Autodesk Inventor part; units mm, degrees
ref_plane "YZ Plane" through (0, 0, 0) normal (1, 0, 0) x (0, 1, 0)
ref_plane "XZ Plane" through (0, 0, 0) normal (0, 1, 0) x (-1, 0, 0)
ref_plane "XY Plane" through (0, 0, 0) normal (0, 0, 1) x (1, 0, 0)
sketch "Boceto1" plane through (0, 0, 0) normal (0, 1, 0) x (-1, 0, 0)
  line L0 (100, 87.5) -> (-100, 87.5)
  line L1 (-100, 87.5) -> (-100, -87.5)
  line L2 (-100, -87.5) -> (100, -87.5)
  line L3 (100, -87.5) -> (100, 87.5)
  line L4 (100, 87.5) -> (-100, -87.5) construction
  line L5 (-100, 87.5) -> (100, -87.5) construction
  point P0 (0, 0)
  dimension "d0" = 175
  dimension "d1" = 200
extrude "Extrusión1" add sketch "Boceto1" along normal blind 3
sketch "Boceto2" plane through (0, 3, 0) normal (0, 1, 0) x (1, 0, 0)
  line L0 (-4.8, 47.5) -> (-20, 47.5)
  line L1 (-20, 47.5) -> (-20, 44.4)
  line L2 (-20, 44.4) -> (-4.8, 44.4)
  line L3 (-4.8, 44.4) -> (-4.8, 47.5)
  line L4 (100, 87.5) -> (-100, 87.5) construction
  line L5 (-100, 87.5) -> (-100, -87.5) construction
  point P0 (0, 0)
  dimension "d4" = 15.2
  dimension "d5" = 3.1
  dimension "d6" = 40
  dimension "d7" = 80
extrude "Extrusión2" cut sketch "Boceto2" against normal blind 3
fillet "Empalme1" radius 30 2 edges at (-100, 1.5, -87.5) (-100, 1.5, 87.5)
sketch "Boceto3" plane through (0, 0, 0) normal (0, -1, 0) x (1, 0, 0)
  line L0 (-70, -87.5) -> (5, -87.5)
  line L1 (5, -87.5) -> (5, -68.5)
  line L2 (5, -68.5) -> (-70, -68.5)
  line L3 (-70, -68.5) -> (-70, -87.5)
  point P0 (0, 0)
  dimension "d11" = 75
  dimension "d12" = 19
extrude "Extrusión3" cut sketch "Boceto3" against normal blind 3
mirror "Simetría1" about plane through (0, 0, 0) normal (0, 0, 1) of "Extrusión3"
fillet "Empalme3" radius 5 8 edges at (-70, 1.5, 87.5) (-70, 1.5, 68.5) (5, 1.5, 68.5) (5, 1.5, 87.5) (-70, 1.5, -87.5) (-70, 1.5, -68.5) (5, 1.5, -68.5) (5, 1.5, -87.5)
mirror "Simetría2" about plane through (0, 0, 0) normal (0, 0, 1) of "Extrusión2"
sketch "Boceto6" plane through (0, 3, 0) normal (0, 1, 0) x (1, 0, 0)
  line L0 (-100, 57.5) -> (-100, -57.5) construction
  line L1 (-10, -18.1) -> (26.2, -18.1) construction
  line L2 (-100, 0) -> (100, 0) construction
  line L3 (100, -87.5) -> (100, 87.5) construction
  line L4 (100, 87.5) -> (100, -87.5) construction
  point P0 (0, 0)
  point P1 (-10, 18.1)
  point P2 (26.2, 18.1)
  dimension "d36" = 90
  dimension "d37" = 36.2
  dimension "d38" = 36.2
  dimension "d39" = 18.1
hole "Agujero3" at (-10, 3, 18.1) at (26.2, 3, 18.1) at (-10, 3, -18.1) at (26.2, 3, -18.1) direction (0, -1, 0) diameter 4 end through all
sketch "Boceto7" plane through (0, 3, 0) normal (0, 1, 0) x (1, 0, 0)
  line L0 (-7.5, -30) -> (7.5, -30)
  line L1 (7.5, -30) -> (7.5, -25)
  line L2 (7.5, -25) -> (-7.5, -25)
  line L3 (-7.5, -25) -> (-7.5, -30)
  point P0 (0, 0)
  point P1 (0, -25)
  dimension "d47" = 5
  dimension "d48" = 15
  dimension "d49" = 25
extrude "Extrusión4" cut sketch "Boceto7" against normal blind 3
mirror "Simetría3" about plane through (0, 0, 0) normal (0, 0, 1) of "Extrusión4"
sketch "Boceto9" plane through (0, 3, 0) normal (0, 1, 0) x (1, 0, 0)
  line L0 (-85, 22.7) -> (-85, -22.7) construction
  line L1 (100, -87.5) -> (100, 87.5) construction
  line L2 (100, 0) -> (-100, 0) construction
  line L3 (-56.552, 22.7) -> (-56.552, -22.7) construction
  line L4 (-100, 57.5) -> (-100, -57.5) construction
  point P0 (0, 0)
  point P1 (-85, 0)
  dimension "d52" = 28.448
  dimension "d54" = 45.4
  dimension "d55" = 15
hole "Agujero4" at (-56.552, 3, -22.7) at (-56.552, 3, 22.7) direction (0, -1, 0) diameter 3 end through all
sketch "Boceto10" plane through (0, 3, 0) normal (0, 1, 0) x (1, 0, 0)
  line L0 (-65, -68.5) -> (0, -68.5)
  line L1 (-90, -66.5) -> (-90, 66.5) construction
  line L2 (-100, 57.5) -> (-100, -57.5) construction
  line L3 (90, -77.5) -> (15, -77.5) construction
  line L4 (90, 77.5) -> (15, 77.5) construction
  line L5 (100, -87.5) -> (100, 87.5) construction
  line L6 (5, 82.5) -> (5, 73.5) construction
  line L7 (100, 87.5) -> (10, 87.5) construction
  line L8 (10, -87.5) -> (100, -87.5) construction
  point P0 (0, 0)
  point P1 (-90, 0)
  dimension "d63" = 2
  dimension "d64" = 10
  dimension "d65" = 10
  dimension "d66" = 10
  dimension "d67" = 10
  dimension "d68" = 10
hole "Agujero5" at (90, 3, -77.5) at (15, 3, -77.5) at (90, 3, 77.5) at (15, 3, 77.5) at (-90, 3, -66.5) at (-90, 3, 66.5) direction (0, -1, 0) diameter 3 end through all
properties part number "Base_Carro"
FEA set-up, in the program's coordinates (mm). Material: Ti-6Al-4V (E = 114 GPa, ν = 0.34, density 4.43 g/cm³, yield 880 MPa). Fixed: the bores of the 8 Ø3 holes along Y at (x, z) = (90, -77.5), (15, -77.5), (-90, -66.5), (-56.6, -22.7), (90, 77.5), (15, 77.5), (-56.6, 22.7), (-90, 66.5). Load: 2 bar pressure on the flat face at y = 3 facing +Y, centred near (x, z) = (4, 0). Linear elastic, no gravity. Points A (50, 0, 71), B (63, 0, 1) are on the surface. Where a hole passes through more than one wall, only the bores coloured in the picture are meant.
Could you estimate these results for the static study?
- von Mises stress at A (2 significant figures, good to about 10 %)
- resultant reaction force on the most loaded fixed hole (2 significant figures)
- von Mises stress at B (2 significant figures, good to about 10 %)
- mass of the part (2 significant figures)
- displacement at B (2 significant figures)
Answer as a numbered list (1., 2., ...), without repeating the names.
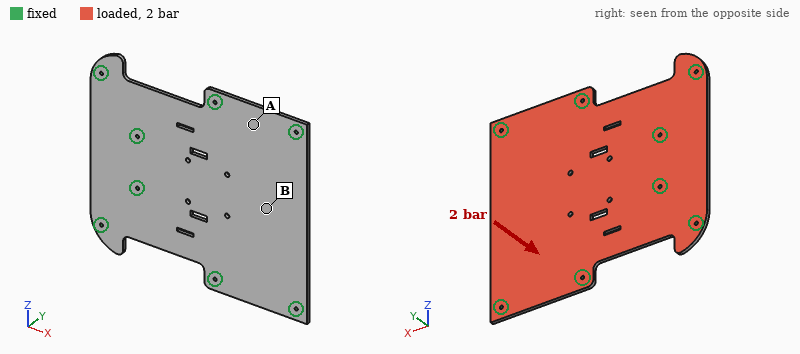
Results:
1. 70 MPa
2. 1.1 kN
3. 130 MPa
4. 420 g
5. 1.5 mm
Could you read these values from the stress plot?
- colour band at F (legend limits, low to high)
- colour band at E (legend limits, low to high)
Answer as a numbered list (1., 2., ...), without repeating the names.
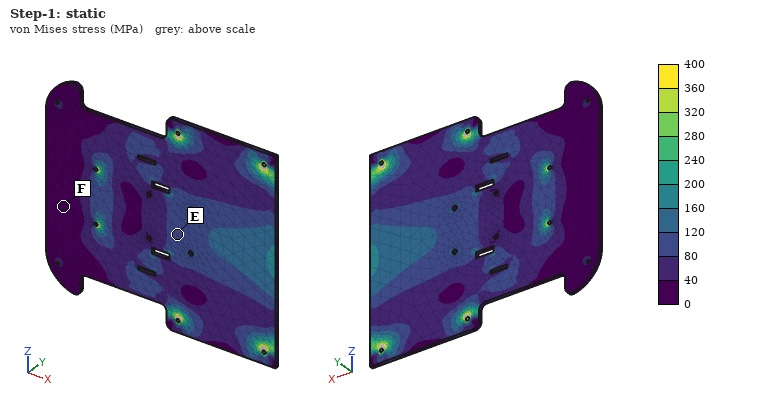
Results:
1. 0 to 40 MPa
2. 80 to 120 MPa
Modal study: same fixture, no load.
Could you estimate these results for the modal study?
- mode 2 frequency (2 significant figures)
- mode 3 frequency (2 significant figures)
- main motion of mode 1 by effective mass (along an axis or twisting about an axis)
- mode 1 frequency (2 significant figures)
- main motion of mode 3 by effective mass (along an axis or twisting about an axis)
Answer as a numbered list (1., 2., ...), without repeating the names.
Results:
1. 1100 Hz
2. 1500 Hz
3. along Y
4. 600 Hz
5. twisting about X
